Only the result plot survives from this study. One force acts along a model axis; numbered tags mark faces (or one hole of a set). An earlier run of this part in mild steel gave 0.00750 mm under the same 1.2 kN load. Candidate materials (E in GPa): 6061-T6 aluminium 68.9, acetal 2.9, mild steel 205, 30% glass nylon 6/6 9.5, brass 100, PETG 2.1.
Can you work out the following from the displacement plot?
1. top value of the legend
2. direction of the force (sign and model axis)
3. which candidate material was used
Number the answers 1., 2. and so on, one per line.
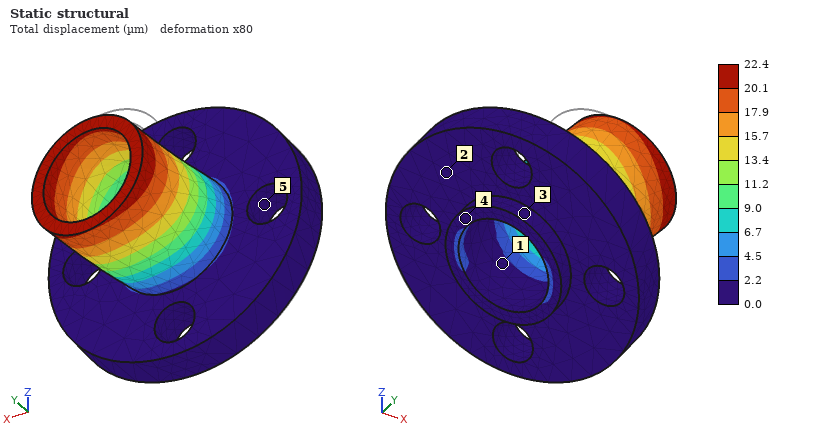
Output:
1. 22.4 µm
2. +X
3. 6061-T6 aluminium
